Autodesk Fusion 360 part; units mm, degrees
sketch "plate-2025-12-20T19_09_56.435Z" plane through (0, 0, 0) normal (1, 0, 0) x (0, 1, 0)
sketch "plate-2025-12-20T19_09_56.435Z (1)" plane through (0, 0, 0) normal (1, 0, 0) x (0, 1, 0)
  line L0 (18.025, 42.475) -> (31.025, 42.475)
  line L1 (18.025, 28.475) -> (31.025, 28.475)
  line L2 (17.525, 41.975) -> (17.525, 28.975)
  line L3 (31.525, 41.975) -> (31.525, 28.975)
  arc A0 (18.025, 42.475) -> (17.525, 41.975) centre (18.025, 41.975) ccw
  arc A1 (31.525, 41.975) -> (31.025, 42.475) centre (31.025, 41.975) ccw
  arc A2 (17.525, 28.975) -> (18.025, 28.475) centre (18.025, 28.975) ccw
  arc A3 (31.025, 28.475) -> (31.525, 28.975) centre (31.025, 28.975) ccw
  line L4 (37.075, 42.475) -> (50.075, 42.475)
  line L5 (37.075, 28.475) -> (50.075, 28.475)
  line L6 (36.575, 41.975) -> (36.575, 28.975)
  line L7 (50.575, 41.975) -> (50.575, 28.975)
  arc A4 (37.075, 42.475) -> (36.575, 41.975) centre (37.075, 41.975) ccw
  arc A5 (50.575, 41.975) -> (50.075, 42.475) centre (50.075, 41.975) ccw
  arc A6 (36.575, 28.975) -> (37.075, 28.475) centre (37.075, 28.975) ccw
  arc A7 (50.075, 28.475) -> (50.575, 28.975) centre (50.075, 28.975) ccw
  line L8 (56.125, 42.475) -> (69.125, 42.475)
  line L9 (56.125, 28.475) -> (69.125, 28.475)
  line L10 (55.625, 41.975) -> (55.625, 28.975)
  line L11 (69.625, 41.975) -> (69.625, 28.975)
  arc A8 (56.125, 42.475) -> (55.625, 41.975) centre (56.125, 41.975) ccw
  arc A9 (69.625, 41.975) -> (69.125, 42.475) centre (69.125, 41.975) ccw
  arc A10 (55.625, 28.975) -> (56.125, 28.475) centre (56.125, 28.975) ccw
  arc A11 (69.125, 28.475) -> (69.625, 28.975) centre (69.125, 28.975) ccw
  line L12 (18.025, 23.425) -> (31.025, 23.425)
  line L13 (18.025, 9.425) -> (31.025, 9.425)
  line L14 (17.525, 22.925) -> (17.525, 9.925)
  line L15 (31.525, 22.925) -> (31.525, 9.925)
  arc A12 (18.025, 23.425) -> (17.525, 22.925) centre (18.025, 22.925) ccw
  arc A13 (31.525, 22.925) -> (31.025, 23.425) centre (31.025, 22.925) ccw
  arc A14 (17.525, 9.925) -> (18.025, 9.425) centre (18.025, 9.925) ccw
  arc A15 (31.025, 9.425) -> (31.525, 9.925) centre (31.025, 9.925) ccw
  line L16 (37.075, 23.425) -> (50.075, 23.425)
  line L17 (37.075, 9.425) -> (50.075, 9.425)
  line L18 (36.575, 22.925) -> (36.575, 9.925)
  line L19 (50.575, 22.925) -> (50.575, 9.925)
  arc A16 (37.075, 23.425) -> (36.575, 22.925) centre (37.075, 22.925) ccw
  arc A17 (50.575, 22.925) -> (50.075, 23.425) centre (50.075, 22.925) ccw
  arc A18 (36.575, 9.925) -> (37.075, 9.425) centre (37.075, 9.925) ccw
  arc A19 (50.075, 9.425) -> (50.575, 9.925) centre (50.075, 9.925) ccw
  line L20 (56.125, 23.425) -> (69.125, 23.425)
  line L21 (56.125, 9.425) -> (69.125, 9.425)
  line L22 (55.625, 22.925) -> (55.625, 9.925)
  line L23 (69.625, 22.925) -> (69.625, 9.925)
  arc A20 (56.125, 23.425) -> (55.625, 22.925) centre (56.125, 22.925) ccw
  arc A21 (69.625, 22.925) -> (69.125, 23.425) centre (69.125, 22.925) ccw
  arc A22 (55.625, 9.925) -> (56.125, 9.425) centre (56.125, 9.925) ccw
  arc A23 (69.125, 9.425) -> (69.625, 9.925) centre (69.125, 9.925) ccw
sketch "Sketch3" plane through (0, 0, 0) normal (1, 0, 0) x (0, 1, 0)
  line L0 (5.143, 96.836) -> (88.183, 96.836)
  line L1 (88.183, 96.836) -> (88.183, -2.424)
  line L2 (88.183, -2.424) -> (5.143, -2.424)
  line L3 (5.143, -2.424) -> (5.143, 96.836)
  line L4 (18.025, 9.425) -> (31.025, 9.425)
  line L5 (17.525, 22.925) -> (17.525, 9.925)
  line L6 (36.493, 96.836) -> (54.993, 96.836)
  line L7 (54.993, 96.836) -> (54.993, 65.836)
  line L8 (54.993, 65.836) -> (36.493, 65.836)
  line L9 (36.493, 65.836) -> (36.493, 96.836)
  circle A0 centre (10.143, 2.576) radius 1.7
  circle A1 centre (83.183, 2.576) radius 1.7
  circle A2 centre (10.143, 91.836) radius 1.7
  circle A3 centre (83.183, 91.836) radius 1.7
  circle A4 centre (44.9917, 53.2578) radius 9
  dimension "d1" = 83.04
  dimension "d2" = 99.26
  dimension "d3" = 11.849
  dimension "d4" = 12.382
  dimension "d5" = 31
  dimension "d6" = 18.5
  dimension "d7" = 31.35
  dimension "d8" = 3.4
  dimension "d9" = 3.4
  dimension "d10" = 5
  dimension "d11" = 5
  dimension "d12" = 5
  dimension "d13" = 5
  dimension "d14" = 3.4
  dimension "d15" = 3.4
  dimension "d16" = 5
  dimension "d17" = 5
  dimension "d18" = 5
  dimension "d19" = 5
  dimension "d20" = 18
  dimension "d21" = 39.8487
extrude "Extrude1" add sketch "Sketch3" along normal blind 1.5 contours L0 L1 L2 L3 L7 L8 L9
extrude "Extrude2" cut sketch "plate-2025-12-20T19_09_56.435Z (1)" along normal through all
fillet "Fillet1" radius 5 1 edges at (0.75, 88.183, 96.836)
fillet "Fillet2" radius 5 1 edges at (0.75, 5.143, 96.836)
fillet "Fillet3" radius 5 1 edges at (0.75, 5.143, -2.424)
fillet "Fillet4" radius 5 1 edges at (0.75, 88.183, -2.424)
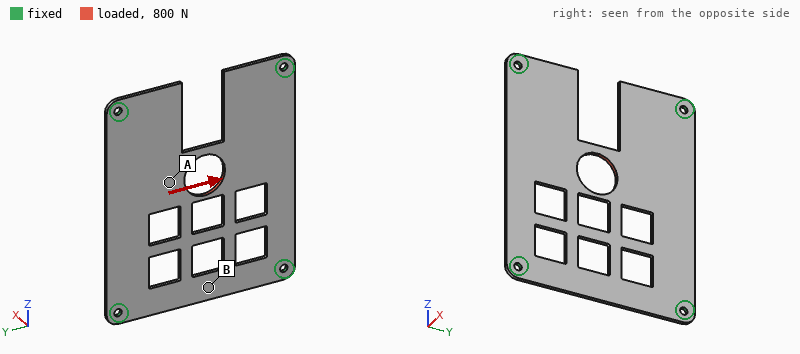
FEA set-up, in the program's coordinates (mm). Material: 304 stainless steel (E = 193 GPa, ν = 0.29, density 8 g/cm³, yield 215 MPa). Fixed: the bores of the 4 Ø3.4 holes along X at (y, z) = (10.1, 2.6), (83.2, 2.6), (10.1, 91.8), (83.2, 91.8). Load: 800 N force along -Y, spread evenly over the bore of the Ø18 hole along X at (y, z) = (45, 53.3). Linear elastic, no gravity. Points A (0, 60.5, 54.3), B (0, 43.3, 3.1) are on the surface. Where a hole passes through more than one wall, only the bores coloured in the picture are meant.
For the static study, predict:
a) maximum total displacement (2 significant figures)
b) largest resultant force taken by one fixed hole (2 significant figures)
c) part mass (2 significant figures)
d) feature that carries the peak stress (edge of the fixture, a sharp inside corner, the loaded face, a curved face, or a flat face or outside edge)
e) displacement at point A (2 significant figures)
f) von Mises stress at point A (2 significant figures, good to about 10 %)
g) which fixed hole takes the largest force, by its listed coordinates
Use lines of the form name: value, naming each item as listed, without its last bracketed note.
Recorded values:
maximum total displacement: 12 µm
largest resultant force taken by one fixed hole: 380 N
part mass: 74 g
feature that carries the peak stress: a curved face
displacement at point A: 9.4 µm
von Mises stress at point A: 10 MPa
which fixed hole takes the largest force, by its listed coordinates: (83.2, 91.8)
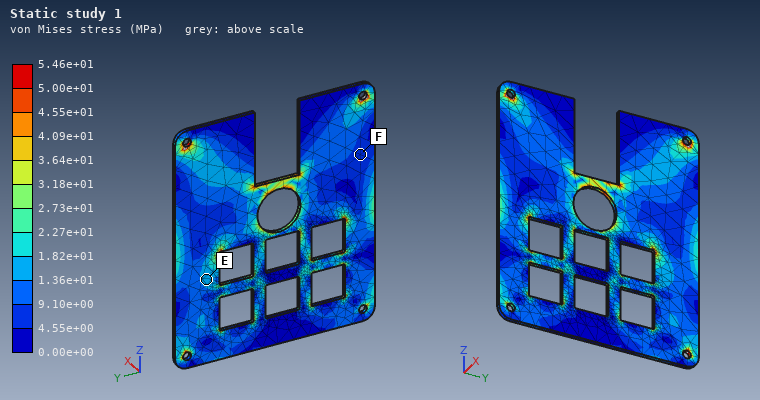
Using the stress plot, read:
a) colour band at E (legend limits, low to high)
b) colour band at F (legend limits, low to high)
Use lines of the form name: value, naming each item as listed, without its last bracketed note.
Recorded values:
colour band at E: 1.36e+01 to 1.82e+01 MPa
colour band at F: 4.55e+00 to 9.10e+00 MPa
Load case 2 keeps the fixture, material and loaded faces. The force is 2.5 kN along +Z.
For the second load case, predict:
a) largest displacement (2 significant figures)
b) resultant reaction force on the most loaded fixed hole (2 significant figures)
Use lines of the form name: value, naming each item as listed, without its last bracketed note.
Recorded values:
largest displacement: 25 µm
resultant reaction force on the most loaded fixed hole: 990 N
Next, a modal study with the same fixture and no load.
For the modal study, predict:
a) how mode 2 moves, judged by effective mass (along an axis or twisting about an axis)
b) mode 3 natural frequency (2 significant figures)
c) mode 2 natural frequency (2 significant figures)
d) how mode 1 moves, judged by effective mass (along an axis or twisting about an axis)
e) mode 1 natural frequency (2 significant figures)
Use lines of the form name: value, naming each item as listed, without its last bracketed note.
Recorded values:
how mode 2 moves, judged by effective mass: twisting about Z
mode 3 natural frequency: 1400 Hz
mode 2 natural frequency: 1100 Hz
how mode 1 moves, judged by effective mass: along X
mode 1 natural frequency: 700 Hz
